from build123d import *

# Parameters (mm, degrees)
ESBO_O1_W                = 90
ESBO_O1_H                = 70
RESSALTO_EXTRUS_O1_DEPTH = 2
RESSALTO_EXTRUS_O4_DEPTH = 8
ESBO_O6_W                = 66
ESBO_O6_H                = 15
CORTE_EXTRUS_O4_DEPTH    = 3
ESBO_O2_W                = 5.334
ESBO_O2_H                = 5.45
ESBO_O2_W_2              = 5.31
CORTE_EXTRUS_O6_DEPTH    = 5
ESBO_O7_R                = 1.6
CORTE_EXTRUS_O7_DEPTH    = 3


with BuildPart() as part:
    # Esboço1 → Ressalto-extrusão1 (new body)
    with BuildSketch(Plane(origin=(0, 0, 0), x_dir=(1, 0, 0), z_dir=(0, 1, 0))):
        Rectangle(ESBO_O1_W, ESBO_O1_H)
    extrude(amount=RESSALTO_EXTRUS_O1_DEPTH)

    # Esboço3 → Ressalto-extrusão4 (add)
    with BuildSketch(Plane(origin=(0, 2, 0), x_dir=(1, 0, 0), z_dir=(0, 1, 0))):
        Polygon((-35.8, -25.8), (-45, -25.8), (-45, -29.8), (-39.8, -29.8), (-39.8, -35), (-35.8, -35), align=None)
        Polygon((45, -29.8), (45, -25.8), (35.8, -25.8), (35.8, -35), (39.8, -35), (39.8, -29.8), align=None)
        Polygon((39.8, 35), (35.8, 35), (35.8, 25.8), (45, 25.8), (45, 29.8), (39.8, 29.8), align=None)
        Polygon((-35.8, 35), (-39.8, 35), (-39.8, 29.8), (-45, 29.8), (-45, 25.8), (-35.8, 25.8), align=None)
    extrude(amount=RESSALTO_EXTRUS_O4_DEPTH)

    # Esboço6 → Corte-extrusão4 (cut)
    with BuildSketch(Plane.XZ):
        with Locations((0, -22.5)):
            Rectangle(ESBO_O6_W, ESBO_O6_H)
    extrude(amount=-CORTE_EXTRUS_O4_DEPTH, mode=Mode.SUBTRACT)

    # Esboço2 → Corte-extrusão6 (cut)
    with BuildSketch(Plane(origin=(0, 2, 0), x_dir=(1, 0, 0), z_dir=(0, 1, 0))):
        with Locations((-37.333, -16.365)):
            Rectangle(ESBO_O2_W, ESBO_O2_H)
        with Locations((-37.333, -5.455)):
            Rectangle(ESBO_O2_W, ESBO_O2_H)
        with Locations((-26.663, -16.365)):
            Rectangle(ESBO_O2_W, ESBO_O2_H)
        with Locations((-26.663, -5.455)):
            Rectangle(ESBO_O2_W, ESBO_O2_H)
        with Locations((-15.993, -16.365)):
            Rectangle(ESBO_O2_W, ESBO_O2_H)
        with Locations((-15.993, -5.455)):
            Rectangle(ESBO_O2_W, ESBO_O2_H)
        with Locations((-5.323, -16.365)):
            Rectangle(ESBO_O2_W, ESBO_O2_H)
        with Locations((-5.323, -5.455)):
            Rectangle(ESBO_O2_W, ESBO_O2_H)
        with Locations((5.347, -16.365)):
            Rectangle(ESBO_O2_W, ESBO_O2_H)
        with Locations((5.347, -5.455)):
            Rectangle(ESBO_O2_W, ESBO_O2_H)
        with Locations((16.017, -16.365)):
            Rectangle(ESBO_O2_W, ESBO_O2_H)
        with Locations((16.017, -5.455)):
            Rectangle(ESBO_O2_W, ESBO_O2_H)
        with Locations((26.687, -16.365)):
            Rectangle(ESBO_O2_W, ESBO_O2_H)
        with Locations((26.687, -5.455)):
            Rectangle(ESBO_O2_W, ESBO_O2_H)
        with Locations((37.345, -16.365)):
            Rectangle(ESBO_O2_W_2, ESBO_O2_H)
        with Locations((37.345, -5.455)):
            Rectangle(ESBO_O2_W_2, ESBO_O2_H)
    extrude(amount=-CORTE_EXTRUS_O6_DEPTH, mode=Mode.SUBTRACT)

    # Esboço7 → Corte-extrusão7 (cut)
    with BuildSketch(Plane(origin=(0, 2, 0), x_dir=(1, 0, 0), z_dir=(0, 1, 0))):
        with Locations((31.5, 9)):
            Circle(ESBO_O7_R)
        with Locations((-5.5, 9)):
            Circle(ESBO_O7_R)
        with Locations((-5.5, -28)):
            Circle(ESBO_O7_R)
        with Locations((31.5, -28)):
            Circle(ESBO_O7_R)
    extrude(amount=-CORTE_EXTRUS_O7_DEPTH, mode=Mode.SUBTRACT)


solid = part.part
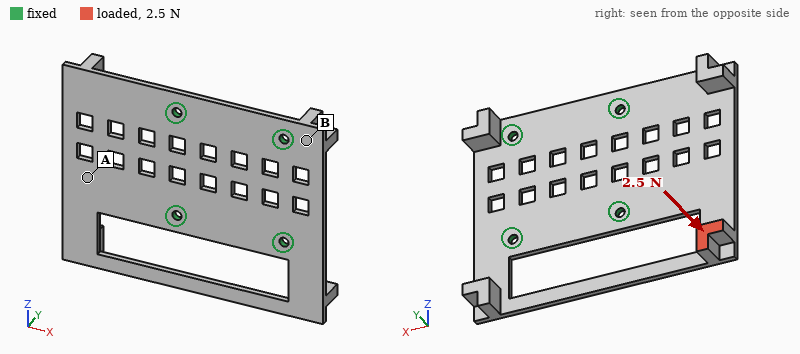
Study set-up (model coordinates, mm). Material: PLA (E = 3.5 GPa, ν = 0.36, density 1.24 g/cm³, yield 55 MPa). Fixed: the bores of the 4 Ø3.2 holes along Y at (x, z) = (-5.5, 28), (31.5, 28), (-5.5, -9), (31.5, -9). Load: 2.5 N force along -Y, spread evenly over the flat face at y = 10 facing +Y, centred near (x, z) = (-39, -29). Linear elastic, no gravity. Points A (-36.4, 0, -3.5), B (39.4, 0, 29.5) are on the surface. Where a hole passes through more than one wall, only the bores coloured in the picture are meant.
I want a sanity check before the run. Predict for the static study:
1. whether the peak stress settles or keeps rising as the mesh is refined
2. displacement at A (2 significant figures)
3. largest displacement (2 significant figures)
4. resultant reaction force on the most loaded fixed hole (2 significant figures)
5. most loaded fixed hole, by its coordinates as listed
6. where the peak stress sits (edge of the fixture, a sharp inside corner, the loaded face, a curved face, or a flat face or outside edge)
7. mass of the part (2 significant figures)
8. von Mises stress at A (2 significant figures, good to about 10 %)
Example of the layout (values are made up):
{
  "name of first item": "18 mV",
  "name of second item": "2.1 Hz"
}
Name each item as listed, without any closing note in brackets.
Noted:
{
  "whether the peak stress settles or keeps rising as the mesh is refined": "keeps rising",
  "displacement at A": "0.37 mm",
  "largest displacement": "1.3 mm",
  "resultant reaction force on the most loaded fixed hole": "3.7 N",
  "most loaded fixed hole, by its coordinates as listed": "(-5.5, -9)",
  "where the peak stress sits": "edge of the fixture",
  "mass of the part": "14 g",
  "von Mises stress at A": "2.6 MPa"
}
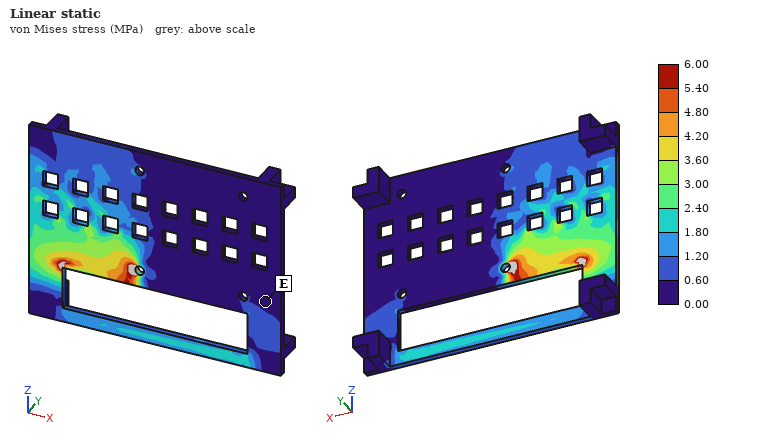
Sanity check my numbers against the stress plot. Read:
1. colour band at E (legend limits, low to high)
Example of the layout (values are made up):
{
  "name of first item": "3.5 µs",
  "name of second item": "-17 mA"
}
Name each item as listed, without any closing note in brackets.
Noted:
{
  "colour band at E": "0.00 to 0.60 MPa"
}
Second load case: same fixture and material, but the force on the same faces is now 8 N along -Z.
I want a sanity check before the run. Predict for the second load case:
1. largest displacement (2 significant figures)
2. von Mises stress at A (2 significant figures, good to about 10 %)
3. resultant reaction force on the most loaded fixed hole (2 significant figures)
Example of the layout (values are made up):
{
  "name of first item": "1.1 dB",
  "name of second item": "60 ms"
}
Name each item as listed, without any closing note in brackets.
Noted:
{
  "largest displacement": "1.3 mm",
  "von Mises stress at A": "2.6 MPa",
  "resultant reaction force on the most loaded fixed hole": "7.3 N"
}
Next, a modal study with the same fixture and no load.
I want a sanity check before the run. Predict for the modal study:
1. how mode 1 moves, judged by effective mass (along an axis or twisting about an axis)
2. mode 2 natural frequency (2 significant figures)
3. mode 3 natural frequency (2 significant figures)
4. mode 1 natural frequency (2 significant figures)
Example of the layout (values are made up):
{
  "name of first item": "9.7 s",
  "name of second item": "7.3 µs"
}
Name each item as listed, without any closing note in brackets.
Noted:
{
  "how mode 1 moves, judged by effective mass": "along Y",
  "mode 2 natural frequency": "300 Hz",
  "mode 3 natural frequency": "410 Hz",
  "mode 1 natural frequency": "200 Hz"
}
